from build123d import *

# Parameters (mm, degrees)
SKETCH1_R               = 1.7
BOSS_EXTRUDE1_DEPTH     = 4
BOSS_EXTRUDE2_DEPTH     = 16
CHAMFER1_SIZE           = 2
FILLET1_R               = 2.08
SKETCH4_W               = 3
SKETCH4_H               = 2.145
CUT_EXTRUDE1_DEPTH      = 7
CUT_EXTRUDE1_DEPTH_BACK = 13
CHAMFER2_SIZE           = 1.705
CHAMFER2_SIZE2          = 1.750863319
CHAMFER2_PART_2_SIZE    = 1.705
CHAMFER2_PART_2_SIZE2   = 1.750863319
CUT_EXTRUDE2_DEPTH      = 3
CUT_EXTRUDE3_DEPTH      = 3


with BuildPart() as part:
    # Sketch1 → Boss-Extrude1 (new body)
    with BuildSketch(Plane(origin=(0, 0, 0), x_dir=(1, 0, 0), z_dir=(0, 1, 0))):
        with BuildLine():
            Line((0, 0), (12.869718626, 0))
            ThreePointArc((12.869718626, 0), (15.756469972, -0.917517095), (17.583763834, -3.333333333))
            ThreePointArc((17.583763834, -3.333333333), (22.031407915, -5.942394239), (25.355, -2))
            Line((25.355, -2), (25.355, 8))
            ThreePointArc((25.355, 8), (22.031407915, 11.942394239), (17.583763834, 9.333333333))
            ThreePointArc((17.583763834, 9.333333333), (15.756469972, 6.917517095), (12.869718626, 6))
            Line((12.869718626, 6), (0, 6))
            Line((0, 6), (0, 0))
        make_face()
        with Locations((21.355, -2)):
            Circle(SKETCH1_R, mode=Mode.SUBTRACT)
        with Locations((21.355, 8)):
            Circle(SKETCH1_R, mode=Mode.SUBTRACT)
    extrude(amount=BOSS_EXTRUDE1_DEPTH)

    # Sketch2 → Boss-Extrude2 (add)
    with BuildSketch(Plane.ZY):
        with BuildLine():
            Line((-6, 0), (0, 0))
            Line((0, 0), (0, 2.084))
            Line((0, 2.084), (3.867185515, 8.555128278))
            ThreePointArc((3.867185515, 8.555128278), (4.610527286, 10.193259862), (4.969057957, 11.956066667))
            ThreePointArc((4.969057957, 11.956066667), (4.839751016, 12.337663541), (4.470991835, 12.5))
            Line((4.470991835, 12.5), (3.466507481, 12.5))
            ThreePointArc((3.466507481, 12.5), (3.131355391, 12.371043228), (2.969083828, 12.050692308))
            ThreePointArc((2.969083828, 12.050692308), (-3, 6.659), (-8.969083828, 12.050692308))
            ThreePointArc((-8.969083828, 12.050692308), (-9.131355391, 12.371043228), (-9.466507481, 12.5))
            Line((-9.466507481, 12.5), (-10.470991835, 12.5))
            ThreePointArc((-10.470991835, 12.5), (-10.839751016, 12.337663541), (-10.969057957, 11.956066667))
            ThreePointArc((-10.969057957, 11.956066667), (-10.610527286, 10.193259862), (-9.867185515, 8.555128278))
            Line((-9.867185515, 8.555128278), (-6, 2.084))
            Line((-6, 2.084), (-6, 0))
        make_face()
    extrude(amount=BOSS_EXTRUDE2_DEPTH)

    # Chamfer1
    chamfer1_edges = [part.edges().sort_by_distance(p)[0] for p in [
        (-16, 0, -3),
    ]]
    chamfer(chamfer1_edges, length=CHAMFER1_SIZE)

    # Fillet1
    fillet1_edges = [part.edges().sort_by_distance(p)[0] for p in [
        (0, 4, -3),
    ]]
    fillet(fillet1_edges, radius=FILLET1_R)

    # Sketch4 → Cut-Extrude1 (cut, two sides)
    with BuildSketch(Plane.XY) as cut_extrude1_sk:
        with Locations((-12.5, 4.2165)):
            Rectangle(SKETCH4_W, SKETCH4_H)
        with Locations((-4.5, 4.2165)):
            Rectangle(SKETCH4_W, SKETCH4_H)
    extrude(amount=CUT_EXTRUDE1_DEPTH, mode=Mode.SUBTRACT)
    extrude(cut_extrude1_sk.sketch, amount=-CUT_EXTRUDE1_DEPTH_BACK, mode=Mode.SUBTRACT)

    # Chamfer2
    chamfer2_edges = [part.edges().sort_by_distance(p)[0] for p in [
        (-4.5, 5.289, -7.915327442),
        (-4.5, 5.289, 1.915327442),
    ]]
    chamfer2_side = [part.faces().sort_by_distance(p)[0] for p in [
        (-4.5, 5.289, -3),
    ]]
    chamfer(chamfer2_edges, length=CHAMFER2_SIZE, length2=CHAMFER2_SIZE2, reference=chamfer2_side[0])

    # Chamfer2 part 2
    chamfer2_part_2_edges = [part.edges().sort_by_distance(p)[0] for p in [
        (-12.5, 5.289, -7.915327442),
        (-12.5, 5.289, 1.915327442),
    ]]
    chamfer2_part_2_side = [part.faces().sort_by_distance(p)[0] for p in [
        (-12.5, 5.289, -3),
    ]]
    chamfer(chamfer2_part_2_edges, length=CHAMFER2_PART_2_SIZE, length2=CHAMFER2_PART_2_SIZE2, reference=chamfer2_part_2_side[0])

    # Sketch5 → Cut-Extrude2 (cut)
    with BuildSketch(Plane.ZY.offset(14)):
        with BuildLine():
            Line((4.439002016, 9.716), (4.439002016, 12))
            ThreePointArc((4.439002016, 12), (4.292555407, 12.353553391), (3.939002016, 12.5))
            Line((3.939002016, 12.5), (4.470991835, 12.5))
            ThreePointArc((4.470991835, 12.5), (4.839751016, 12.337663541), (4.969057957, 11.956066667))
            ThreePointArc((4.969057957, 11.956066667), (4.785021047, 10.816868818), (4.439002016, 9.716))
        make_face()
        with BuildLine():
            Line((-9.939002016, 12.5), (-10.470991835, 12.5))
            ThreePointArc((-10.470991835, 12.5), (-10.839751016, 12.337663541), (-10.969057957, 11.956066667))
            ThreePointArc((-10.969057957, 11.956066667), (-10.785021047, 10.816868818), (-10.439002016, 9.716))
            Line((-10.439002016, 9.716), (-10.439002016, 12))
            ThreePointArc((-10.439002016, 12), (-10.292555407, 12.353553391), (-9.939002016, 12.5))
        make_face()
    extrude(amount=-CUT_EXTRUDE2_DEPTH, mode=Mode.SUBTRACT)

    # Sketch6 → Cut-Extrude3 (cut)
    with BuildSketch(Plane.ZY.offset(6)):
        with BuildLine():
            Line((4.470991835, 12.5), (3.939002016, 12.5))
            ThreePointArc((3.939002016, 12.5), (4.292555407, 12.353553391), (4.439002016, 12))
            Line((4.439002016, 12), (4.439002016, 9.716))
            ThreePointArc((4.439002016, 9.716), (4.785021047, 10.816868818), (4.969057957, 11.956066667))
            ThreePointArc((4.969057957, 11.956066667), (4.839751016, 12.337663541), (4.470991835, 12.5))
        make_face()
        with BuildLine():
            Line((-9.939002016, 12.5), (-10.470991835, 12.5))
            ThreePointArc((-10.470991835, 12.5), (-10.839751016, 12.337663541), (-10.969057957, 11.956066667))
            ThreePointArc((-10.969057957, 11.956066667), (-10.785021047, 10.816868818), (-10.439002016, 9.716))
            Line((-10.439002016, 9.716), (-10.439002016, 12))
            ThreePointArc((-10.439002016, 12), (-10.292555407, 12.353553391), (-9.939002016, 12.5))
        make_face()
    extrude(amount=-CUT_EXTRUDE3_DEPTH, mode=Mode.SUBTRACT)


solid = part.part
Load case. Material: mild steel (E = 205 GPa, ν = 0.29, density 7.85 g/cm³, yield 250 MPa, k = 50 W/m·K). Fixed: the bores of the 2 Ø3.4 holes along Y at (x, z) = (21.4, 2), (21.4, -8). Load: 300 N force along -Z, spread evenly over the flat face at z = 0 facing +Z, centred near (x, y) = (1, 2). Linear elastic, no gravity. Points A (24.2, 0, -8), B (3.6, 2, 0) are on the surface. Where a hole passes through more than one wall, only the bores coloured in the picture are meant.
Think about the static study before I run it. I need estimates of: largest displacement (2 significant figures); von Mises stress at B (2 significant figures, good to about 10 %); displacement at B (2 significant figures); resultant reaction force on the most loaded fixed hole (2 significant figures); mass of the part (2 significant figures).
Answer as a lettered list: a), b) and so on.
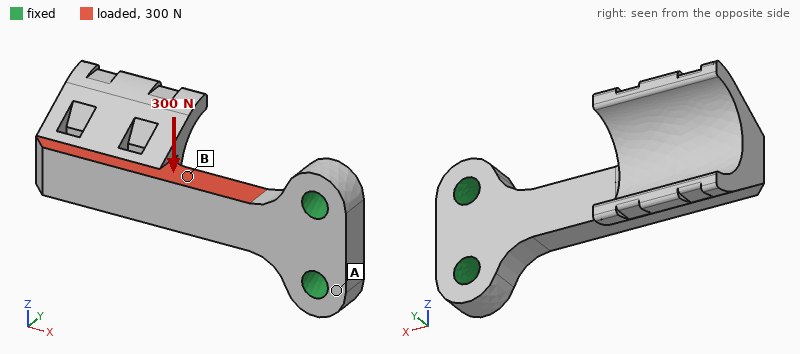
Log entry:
a) 78 µm
b) 57 MPa
c) 23 µm
d) 600 N
e) 16 g
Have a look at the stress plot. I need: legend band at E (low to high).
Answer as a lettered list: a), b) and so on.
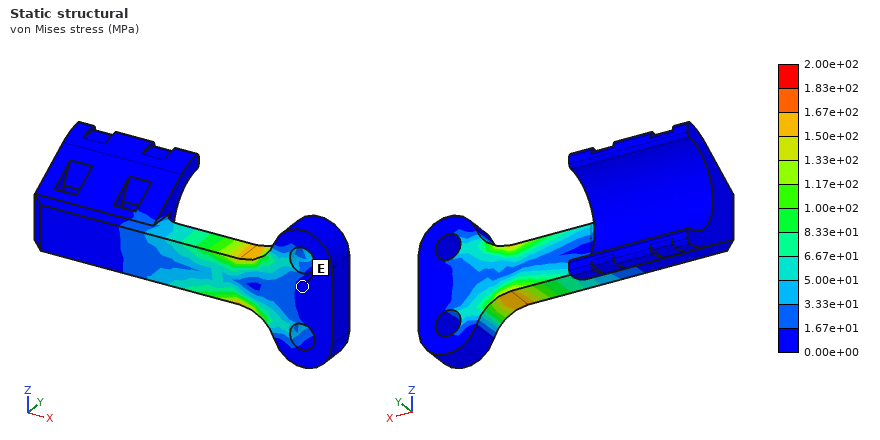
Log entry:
a) 0.00e+00 to 1.67e+01 MPa
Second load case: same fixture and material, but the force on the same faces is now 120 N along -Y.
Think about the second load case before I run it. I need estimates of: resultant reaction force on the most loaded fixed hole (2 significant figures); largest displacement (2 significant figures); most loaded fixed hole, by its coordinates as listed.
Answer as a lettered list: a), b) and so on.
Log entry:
a) 99 N
b) 0.10 mm
c) (21.4, 2)
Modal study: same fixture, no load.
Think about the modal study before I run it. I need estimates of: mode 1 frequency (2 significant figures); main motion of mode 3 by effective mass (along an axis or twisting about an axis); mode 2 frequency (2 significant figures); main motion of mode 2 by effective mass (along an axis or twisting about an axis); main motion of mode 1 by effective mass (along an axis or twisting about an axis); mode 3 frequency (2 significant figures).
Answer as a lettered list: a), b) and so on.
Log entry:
a) 1600 Hz
b) twisting about X
c) 2500 Hz
d) along Z
e) along Y
f) 5800 Hz
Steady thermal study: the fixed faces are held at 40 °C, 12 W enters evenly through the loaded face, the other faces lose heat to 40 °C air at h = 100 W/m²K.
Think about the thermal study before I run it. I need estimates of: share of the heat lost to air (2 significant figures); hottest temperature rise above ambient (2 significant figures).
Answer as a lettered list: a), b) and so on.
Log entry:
a) 54 %
b) 59 K
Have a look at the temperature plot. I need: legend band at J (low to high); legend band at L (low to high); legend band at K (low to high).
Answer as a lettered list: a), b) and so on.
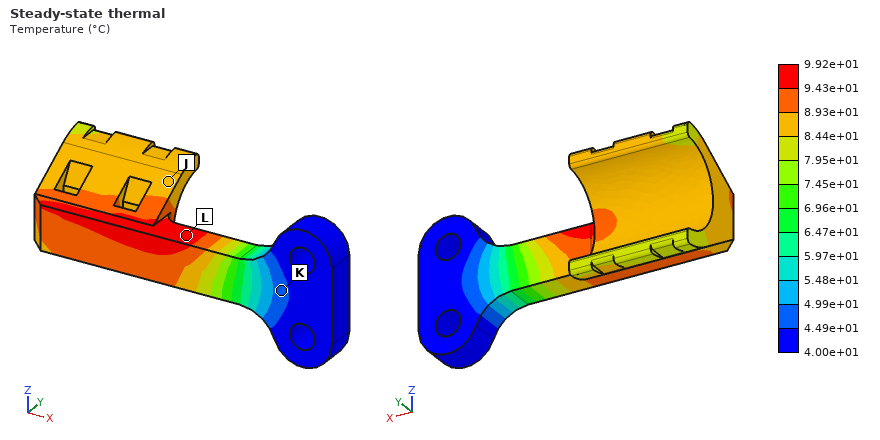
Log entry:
a) 8.44e+01 to 8.93e+01 °C
b) 9.43e+01 to 9.92e+01 °C
c) 4.49e+01 to 4.99e+01 °C
